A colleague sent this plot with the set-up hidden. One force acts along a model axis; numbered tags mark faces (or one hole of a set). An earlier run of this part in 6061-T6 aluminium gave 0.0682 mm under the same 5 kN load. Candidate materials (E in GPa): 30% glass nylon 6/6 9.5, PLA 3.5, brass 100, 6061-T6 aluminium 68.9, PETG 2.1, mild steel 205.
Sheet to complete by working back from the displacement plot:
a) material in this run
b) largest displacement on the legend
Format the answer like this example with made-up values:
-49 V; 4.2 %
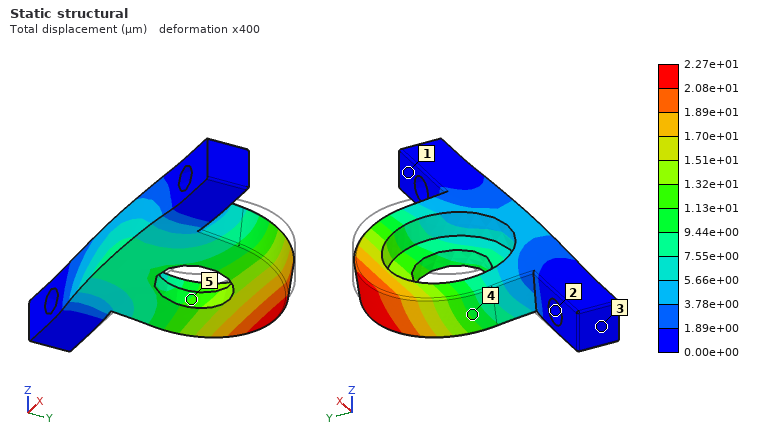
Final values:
mild steel; 2.27e+01 µm
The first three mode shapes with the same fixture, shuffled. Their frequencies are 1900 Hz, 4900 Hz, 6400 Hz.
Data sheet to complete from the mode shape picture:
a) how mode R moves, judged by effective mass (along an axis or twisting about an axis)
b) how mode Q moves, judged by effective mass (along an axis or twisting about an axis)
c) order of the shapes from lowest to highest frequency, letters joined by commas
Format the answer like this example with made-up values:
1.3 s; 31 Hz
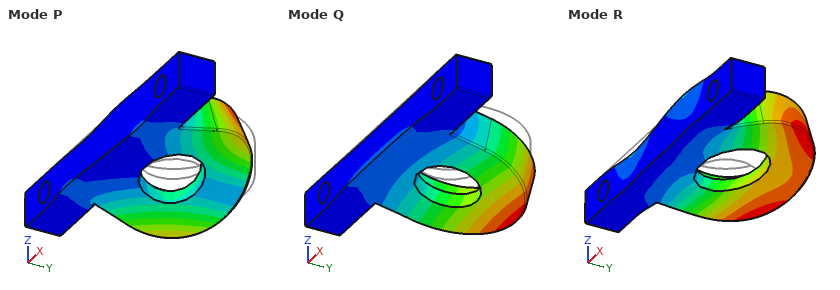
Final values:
along X; along Z; Q, P, R
